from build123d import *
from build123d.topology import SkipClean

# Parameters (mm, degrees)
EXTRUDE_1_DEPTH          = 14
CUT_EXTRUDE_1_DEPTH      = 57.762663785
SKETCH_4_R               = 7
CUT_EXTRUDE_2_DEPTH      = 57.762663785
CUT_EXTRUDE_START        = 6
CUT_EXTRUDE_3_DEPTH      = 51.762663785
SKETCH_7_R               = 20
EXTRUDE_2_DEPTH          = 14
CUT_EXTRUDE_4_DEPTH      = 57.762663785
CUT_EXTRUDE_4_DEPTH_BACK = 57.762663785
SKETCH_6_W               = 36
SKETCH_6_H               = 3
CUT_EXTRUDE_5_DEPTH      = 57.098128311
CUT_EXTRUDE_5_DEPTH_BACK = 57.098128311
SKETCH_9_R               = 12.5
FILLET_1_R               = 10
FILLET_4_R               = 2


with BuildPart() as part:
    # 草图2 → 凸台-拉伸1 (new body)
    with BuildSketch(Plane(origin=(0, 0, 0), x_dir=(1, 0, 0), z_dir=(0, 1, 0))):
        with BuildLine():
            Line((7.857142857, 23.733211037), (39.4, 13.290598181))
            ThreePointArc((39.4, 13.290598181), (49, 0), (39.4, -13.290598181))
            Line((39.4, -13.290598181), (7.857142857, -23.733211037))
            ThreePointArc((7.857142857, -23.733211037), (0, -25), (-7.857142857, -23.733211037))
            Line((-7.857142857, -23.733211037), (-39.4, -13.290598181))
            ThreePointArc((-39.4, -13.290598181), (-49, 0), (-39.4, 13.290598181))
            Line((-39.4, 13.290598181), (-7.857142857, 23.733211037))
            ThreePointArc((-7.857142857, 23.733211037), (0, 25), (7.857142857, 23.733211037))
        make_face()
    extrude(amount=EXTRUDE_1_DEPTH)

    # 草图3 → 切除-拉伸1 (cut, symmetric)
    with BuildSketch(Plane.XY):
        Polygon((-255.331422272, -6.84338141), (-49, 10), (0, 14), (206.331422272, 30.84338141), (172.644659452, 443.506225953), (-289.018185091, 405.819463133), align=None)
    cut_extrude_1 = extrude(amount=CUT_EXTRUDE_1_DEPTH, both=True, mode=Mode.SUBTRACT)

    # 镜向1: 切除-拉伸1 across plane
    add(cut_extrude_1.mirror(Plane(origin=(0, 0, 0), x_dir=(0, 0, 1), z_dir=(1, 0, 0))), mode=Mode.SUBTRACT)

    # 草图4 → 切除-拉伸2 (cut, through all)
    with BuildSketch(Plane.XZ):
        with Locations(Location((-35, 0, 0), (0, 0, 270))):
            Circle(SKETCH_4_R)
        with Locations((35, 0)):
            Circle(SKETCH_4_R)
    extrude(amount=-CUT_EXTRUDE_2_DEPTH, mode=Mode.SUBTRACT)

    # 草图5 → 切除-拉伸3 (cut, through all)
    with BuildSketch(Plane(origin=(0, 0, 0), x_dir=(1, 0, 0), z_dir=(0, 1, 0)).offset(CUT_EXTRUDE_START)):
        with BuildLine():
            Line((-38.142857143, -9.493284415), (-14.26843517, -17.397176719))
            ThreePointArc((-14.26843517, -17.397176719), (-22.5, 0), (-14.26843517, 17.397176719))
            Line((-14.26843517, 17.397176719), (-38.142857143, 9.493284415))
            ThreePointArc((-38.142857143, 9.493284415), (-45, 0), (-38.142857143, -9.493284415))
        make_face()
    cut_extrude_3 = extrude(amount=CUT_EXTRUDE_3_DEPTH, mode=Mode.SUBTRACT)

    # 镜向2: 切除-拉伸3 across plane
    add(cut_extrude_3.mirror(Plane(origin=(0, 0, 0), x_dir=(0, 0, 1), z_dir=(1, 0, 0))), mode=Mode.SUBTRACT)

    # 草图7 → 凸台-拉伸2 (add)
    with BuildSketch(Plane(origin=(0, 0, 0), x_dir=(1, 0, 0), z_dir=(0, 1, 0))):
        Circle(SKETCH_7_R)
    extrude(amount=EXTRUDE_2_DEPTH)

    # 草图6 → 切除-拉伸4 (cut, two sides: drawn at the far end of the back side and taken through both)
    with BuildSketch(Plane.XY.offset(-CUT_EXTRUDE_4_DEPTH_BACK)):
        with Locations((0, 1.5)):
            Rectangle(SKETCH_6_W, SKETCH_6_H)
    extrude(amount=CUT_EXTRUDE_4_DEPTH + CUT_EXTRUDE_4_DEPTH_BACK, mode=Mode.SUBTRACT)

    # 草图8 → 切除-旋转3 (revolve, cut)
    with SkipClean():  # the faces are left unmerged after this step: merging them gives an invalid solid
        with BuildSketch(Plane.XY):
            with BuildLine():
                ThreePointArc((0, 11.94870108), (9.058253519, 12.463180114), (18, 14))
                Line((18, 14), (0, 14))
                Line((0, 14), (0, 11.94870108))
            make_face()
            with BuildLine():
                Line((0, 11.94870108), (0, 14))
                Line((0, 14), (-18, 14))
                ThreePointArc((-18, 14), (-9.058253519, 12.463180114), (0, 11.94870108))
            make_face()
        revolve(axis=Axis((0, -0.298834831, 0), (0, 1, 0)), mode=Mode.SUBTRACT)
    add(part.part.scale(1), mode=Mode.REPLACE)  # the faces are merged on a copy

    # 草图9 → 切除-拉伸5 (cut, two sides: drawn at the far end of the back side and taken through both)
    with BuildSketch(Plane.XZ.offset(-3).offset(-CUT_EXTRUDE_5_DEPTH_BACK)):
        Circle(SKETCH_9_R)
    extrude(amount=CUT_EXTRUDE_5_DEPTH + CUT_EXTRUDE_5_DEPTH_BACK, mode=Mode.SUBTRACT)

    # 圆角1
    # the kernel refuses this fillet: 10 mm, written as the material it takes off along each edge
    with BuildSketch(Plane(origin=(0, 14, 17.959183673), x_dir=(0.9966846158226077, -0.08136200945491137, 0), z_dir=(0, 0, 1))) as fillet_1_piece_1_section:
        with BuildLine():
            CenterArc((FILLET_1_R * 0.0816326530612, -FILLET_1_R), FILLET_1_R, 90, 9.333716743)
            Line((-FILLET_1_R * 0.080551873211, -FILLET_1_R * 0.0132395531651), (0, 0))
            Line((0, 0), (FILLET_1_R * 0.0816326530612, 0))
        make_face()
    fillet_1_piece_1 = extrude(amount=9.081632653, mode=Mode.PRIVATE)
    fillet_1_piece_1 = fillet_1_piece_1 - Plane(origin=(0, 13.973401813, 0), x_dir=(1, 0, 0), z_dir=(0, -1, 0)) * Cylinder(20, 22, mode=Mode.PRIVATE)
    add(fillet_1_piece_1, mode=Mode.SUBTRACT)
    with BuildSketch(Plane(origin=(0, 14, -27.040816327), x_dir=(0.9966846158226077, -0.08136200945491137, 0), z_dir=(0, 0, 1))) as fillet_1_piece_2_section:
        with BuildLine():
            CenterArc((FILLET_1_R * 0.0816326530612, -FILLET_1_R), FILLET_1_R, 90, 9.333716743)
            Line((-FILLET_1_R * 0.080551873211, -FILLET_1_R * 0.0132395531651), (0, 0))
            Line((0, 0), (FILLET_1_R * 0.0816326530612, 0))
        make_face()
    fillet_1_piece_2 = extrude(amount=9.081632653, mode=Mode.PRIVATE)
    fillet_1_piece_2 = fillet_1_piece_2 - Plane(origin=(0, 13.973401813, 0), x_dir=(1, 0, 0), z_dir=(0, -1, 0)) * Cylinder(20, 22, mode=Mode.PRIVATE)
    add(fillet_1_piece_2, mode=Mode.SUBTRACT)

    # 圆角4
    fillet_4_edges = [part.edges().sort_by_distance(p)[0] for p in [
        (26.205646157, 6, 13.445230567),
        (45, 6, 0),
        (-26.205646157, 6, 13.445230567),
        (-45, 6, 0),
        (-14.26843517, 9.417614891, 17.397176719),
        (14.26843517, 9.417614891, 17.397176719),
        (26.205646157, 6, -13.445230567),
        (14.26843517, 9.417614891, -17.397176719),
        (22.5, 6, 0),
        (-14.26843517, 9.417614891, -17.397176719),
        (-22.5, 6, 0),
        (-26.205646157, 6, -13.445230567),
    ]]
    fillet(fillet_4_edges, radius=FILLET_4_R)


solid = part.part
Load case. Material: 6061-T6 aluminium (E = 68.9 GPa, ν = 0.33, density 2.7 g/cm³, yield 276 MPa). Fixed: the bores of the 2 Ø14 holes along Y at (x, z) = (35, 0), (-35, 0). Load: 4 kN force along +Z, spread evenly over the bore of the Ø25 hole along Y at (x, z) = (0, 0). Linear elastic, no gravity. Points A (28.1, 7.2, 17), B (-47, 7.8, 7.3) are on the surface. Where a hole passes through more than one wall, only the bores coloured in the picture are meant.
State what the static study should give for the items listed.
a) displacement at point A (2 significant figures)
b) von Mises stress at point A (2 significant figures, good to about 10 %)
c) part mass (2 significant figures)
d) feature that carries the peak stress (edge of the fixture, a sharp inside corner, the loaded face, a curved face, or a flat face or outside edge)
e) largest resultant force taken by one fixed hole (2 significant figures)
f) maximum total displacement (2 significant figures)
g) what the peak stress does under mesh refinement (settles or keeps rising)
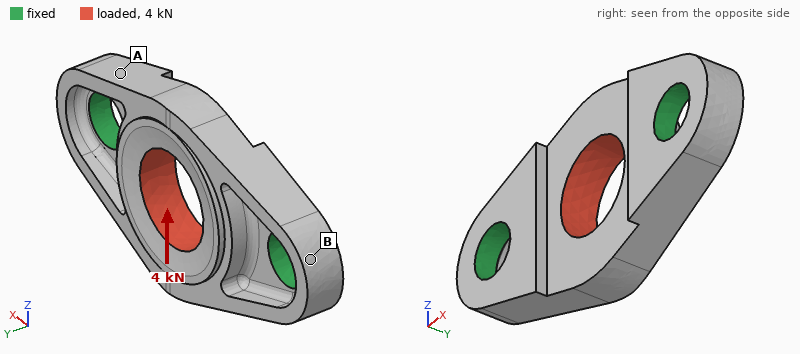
10 µm
14 MPa
70 g
edge of the fixture
2.0 kN
33 µm
keeps rising
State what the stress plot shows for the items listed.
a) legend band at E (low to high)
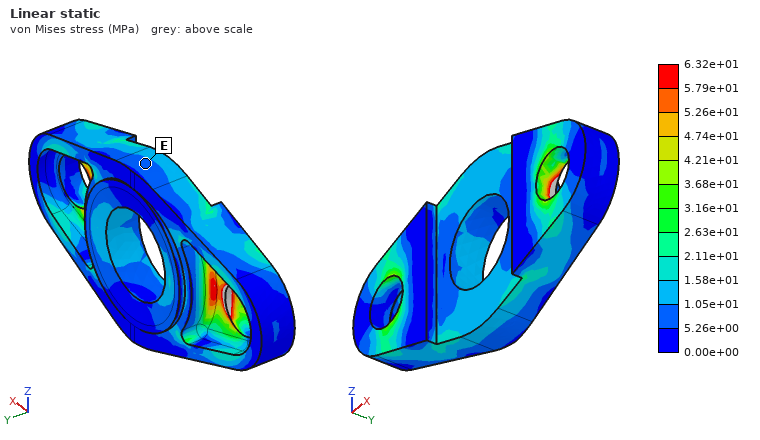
5.26e+00 to 1.05e+01 MPa
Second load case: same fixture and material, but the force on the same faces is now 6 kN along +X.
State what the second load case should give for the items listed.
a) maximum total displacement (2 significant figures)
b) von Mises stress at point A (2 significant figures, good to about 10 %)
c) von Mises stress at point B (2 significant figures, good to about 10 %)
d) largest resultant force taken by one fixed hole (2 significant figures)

8.6 µm
8.3 MPa
3.4 MPa
3.0 kN
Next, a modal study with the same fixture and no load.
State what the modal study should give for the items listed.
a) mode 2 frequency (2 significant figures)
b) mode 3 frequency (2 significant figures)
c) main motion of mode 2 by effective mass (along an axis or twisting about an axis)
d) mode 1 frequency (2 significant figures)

9100 Hz
18 kHz
along Y
6800 Hz
